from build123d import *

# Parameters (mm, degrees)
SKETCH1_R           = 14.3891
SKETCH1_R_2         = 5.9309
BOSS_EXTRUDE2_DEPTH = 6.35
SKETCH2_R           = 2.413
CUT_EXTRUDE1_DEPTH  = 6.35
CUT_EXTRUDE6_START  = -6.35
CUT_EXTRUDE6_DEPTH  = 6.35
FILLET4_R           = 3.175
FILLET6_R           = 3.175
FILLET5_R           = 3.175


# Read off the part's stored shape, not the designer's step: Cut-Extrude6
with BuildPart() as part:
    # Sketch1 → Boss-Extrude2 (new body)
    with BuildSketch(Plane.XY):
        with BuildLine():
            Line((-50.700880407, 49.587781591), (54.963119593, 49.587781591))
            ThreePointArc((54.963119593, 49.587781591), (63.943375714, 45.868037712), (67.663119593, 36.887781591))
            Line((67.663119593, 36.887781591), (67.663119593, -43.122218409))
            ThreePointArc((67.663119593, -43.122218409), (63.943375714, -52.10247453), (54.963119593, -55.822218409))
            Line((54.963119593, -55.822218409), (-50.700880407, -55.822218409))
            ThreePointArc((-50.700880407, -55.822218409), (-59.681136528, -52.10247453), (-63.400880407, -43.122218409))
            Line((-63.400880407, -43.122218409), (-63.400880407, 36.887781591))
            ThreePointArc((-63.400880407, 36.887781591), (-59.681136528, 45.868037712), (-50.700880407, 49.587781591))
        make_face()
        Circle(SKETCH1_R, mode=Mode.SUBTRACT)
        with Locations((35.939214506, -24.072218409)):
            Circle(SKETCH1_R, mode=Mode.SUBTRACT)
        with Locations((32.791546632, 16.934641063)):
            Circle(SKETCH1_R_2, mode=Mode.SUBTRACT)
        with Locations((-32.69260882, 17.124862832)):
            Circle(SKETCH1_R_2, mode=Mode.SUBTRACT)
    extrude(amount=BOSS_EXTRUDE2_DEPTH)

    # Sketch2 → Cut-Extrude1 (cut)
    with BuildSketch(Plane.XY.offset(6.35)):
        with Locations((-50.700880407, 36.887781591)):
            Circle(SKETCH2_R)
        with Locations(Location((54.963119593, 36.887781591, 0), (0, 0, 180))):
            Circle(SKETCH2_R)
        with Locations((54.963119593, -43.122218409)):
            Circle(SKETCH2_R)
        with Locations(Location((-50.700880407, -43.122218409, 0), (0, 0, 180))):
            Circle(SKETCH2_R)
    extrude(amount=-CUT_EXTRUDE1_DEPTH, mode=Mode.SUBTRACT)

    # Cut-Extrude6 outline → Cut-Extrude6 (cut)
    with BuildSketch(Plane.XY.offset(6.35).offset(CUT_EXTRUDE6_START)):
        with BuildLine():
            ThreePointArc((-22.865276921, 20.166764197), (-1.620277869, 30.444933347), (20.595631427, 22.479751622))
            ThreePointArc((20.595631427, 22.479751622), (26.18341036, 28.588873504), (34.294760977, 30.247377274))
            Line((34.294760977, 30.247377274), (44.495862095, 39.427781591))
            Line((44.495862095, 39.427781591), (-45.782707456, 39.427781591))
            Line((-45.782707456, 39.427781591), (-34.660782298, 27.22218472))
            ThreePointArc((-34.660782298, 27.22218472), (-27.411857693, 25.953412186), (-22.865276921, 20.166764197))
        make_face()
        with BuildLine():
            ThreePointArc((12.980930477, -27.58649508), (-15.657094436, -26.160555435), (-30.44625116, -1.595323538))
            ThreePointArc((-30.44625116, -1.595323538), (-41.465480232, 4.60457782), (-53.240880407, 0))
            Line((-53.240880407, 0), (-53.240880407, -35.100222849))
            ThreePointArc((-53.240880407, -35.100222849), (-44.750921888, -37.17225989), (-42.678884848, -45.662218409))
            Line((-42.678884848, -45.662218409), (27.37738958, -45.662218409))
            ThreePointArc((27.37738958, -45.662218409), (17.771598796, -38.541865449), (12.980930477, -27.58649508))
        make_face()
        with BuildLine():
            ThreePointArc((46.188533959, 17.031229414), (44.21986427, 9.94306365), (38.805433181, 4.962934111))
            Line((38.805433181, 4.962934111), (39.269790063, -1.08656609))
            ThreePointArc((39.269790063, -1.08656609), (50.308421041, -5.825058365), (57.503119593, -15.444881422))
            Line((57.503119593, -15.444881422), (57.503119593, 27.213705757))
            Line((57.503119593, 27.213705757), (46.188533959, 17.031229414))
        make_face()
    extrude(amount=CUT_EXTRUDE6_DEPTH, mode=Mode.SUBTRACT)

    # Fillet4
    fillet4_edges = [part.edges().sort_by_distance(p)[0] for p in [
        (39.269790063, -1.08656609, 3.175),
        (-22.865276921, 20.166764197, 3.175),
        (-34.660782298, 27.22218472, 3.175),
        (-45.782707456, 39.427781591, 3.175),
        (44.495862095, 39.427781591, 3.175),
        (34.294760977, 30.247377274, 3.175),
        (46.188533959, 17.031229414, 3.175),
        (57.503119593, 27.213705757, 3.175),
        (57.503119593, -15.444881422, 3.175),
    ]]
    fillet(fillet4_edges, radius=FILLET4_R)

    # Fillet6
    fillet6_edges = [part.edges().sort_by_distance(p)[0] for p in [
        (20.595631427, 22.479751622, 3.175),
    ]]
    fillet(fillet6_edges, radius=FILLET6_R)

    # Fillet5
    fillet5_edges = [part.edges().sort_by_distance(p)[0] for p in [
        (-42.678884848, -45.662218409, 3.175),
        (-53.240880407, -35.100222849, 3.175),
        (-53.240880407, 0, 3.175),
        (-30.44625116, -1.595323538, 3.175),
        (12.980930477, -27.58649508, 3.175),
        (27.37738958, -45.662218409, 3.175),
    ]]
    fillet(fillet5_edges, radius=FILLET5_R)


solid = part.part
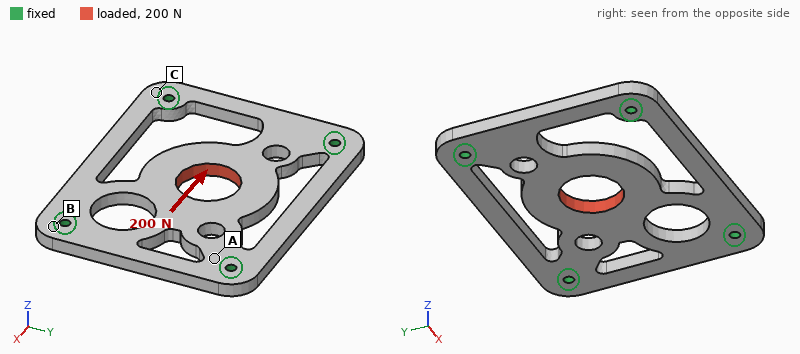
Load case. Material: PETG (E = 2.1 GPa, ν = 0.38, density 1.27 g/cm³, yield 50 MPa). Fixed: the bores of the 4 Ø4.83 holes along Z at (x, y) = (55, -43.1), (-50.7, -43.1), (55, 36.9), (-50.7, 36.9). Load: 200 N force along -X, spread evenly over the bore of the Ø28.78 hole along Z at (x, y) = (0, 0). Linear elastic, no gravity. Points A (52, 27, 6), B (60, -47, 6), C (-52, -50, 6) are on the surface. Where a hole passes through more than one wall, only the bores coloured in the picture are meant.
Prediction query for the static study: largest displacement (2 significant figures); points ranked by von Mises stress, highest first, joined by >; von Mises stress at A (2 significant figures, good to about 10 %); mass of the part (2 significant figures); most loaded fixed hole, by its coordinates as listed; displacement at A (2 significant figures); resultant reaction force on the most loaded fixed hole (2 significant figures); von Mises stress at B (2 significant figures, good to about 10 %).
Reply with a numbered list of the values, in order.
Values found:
1. 43 µm
2. A > B > C
3. 0.90 MPa
4. 71 g
5. (55, 36.9)
6. 7.7 µm
7. 92 N
8. 0.48 MPa
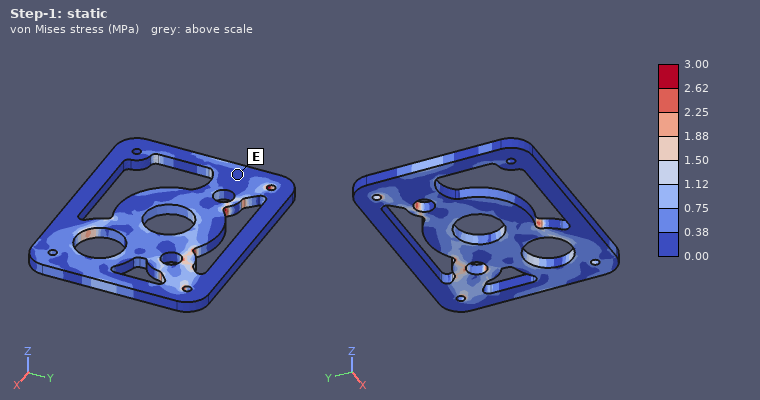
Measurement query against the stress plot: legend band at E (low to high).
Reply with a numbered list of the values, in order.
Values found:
1. 0.00 to 0.38 MPa
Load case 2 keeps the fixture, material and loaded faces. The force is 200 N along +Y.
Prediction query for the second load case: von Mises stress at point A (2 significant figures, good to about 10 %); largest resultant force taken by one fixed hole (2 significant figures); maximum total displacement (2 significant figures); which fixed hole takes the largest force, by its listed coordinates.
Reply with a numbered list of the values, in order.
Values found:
1. 0.86 MPa
2. 110 N
3. 60 µm
4. (55, 36.9)
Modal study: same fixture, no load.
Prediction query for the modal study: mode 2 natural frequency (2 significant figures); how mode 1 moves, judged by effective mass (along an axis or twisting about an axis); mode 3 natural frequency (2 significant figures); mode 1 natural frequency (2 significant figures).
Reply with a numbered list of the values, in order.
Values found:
1. 780 Hz
2. along Z
3. 840 Hz
4. 470 Hz
